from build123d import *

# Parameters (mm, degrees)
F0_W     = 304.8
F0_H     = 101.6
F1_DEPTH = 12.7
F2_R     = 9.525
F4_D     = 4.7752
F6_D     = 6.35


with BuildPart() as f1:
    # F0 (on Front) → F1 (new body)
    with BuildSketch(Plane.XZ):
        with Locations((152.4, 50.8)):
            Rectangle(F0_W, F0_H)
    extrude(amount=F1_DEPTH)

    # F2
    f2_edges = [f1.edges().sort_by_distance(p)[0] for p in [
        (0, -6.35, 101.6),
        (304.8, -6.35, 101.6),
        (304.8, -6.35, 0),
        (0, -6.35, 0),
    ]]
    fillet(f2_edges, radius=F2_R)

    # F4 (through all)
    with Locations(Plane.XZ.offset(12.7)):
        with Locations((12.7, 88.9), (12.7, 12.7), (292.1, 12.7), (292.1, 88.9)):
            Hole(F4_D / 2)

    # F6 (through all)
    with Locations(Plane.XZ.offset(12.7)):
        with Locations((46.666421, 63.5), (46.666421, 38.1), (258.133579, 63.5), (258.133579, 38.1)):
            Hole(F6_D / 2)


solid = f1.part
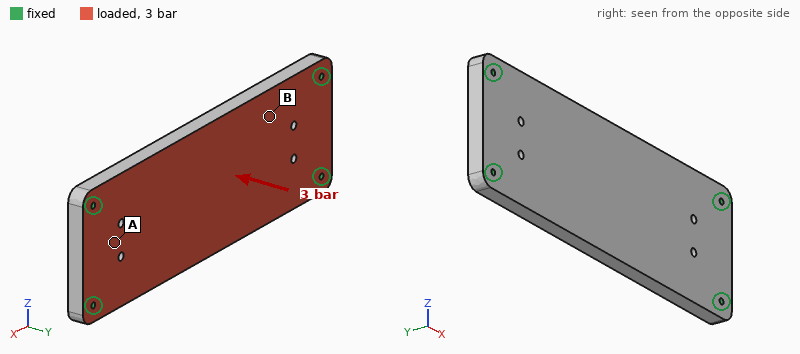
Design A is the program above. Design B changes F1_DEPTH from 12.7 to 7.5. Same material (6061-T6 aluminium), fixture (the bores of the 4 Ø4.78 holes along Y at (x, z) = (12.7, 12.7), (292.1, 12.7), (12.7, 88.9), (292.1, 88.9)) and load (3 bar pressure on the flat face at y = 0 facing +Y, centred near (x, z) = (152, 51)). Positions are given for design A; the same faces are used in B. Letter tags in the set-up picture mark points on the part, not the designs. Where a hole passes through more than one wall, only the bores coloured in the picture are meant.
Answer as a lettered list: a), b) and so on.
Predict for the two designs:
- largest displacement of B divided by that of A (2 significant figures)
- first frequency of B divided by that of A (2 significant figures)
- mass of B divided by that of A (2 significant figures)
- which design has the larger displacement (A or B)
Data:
a) 4.5
b) 0.62
c) 0.59
d) B
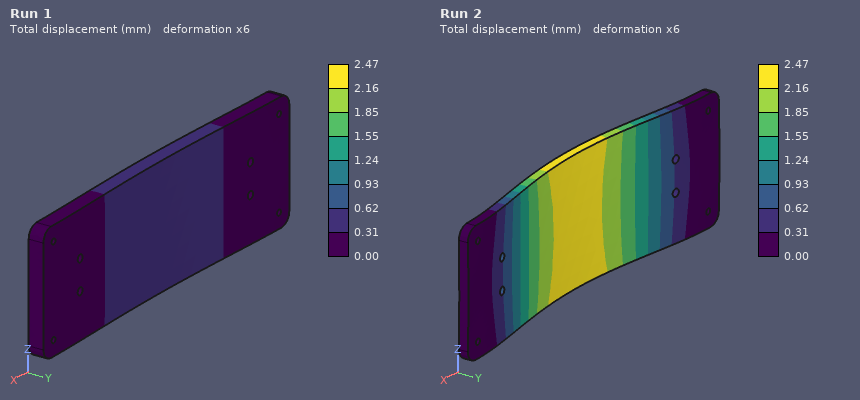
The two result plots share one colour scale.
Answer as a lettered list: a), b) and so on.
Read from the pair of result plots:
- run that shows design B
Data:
a) Run 2
